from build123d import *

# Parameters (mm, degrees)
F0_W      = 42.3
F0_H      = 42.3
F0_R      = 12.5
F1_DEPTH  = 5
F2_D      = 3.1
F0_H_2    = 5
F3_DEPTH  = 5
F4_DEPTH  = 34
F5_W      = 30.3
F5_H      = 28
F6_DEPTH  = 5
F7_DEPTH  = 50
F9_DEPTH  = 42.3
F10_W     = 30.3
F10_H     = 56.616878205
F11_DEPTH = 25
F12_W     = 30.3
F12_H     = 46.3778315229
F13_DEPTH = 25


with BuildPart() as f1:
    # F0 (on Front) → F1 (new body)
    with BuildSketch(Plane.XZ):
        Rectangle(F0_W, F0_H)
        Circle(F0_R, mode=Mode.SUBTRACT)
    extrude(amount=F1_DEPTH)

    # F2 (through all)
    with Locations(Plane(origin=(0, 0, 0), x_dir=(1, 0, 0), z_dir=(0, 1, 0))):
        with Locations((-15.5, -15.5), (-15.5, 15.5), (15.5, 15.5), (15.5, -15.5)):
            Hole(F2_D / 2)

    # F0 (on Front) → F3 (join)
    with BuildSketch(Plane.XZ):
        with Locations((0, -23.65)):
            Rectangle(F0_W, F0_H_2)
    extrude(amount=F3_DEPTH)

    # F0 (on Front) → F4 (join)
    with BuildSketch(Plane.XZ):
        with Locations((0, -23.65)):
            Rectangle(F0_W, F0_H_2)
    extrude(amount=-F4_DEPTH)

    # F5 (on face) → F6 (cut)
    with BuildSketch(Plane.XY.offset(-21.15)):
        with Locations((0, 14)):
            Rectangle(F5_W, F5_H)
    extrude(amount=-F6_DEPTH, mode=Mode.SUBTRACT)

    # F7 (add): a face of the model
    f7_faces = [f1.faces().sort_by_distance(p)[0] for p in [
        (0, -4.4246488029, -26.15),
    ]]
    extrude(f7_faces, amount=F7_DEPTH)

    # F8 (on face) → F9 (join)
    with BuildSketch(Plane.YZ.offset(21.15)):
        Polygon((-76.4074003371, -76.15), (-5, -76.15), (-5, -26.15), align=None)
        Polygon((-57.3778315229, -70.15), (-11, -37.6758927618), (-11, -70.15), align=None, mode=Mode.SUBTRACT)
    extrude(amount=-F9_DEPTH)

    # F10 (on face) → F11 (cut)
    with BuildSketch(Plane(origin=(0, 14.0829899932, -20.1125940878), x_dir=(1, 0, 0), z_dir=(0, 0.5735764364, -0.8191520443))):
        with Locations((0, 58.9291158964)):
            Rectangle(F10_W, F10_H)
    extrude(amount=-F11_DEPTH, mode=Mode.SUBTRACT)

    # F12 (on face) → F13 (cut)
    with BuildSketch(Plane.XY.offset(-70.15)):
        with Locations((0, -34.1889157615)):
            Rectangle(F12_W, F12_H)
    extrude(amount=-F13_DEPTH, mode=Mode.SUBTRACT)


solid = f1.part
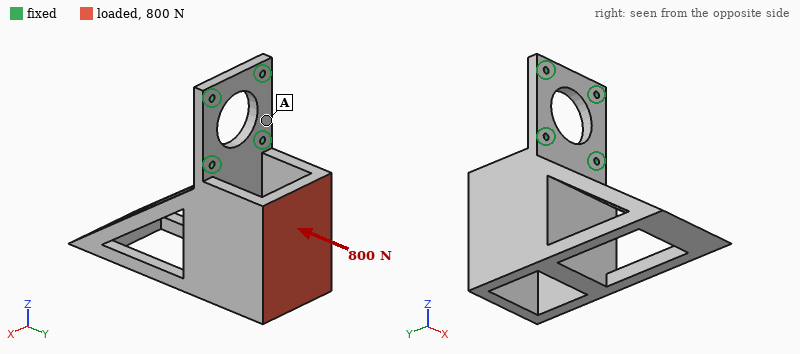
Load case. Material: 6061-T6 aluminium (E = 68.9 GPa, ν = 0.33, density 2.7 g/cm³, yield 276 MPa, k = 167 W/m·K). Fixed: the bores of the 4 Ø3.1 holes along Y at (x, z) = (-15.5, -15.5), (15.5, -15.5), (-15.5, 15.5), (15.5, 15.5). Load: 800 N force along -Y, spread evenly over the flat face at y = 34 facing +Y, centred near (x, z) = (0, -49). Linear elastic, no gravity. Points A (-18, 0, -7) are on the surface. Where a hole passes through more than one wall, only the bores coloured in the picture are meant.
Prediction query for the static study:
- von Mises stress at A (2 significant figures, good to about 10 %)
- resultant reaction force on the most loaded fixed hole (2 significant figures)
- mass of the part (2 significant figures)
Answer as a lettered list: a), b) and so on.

a) 21 MPa
b) 490 N
c) 200 g
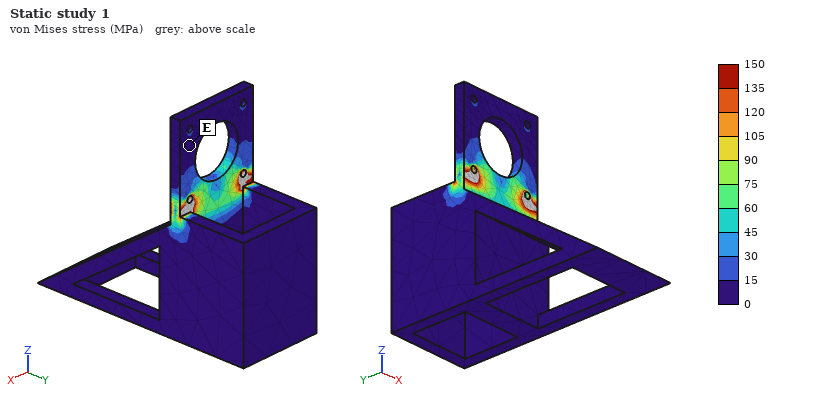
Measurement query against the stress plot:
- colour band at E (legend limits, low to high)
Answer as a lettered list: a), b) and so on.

a) 0 to 15 MPa
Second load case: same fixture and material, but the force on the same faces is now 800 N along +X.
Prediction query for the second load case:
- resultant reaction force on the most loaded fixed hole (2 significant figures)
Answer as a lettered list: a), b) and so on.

a) 1.2 kN
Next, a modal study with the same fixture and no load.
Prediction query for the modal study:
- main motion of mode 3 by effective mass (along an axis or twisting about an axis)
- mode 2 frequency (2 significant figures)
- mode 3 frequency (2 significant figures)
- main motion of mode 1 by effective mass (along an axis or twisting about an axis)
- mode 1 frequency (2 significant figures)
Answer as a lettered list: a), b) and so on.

a) along X
b) 1300 Hz
c) 2200 Hz
d) along Y
e) 400 Hz
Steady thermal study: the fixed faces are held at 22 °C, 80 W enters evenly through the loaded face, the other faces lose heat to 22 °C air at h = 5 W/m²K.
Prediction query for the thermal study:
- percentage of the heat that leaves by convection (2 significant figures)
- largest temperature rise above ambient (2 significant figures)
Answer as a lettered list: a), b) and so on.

a) 6.4 %
b) 67 K
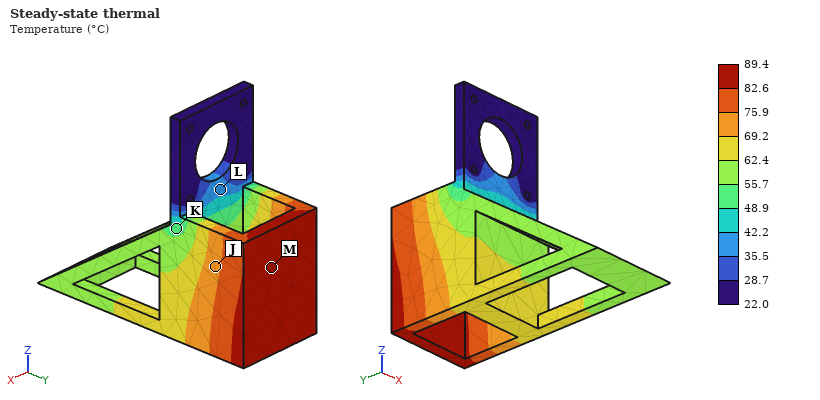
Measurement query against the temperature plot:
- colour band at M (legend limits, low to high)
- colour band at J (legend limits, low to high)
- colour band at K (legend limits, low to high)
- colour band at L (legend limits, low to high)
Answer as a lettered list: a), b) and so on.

a) 82.6 to 89.4 °C
b) 69.2 to 75.9 °C
c) 48.9 to 55.7 °C
d) 35.5 to 42.2 °C
